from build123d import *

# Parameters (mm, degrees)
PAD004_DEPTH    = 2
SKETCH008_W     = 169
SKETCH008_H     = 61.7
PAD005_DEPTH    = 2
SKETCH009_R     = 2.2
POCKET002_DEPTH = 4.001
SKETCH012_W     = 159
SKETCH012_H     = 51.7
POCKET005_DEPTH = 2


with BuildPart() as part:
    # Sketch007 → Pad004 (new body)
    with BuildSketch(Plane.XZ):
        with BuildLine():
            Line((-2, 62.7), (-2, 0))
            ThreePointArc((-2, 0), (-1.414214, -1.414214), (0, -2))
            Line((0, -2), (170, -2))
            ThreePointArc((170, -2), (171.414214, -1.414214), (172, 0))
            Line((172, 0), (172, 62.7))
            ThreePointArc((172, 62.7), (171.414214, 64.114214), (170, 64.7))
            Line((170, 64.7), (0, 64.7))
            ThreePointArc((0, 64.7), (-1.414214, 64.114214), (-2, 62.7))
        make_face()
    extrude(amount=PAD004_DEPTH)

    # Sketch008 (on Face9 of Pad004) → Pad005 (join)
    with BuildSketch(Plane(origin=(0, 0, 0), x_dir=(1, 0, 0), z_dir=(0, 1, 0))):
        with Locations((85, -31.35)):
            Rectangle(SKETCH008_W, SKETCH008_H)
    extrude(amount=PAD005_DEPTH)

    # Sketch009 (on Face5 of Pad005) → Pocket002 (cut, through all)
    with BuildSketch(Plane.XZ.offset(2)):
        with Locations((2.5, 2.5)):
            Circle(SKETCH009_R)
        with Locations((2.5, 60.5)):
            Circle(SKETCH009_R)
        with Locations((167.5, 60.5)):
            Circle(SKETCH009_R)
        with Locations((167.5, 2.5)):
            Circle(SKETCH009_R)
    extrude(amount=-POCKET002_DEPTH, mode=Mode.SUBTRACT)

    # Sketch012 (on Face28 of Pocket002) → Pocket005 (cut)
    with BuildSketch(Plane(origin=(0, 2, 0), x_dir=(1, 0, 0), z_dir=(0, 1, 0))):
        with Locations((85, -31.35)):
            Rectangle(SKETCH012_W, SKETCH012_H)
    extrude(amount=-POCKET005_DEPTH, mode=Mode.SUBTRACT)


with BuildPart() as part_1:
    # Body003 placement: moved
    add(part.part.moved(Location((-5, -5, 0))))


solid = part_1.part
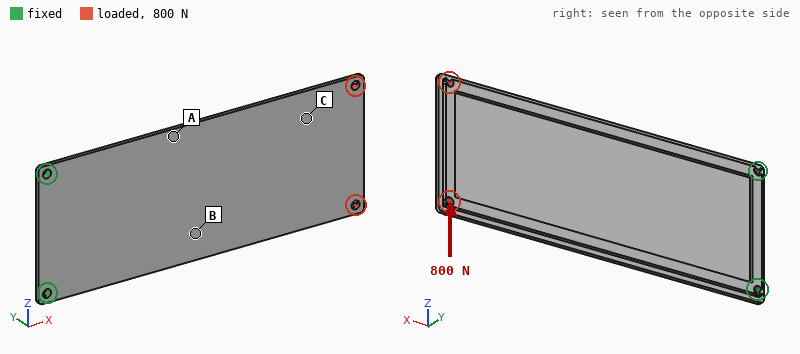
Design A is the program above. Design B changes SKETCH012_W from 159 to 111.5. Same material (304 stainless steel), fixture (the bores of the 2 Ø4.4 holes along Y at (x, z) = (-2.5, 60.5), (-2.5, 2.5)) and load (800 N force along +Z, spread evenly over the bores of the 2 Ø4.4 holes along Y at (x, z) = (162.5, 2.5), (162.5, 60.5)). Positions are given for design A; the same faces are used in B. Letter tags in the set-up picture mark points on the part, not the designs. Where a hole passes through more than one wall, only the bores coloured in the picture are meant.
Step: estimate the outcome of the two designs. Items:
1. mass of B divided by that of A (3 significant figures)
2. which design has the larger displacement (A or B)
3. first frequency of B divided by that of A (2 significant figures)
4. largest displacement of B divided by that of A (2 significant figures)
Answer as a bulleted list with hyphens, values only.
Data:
- 1.18
- A
- 1.0
- 0.77
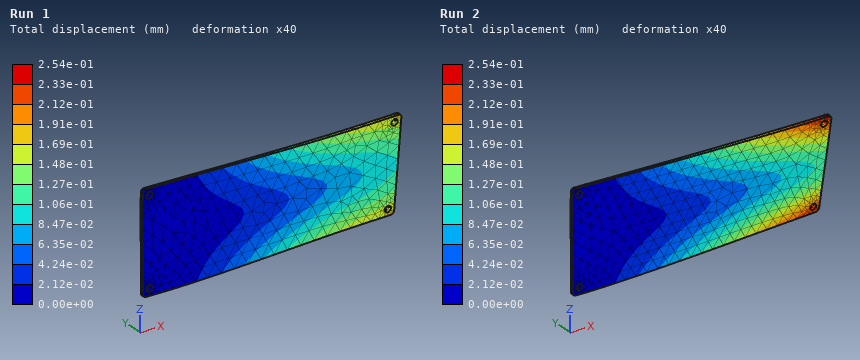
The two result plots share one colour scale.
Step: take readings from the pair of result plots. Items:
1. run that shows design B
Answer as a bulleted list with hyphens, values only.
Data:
- Run 1
